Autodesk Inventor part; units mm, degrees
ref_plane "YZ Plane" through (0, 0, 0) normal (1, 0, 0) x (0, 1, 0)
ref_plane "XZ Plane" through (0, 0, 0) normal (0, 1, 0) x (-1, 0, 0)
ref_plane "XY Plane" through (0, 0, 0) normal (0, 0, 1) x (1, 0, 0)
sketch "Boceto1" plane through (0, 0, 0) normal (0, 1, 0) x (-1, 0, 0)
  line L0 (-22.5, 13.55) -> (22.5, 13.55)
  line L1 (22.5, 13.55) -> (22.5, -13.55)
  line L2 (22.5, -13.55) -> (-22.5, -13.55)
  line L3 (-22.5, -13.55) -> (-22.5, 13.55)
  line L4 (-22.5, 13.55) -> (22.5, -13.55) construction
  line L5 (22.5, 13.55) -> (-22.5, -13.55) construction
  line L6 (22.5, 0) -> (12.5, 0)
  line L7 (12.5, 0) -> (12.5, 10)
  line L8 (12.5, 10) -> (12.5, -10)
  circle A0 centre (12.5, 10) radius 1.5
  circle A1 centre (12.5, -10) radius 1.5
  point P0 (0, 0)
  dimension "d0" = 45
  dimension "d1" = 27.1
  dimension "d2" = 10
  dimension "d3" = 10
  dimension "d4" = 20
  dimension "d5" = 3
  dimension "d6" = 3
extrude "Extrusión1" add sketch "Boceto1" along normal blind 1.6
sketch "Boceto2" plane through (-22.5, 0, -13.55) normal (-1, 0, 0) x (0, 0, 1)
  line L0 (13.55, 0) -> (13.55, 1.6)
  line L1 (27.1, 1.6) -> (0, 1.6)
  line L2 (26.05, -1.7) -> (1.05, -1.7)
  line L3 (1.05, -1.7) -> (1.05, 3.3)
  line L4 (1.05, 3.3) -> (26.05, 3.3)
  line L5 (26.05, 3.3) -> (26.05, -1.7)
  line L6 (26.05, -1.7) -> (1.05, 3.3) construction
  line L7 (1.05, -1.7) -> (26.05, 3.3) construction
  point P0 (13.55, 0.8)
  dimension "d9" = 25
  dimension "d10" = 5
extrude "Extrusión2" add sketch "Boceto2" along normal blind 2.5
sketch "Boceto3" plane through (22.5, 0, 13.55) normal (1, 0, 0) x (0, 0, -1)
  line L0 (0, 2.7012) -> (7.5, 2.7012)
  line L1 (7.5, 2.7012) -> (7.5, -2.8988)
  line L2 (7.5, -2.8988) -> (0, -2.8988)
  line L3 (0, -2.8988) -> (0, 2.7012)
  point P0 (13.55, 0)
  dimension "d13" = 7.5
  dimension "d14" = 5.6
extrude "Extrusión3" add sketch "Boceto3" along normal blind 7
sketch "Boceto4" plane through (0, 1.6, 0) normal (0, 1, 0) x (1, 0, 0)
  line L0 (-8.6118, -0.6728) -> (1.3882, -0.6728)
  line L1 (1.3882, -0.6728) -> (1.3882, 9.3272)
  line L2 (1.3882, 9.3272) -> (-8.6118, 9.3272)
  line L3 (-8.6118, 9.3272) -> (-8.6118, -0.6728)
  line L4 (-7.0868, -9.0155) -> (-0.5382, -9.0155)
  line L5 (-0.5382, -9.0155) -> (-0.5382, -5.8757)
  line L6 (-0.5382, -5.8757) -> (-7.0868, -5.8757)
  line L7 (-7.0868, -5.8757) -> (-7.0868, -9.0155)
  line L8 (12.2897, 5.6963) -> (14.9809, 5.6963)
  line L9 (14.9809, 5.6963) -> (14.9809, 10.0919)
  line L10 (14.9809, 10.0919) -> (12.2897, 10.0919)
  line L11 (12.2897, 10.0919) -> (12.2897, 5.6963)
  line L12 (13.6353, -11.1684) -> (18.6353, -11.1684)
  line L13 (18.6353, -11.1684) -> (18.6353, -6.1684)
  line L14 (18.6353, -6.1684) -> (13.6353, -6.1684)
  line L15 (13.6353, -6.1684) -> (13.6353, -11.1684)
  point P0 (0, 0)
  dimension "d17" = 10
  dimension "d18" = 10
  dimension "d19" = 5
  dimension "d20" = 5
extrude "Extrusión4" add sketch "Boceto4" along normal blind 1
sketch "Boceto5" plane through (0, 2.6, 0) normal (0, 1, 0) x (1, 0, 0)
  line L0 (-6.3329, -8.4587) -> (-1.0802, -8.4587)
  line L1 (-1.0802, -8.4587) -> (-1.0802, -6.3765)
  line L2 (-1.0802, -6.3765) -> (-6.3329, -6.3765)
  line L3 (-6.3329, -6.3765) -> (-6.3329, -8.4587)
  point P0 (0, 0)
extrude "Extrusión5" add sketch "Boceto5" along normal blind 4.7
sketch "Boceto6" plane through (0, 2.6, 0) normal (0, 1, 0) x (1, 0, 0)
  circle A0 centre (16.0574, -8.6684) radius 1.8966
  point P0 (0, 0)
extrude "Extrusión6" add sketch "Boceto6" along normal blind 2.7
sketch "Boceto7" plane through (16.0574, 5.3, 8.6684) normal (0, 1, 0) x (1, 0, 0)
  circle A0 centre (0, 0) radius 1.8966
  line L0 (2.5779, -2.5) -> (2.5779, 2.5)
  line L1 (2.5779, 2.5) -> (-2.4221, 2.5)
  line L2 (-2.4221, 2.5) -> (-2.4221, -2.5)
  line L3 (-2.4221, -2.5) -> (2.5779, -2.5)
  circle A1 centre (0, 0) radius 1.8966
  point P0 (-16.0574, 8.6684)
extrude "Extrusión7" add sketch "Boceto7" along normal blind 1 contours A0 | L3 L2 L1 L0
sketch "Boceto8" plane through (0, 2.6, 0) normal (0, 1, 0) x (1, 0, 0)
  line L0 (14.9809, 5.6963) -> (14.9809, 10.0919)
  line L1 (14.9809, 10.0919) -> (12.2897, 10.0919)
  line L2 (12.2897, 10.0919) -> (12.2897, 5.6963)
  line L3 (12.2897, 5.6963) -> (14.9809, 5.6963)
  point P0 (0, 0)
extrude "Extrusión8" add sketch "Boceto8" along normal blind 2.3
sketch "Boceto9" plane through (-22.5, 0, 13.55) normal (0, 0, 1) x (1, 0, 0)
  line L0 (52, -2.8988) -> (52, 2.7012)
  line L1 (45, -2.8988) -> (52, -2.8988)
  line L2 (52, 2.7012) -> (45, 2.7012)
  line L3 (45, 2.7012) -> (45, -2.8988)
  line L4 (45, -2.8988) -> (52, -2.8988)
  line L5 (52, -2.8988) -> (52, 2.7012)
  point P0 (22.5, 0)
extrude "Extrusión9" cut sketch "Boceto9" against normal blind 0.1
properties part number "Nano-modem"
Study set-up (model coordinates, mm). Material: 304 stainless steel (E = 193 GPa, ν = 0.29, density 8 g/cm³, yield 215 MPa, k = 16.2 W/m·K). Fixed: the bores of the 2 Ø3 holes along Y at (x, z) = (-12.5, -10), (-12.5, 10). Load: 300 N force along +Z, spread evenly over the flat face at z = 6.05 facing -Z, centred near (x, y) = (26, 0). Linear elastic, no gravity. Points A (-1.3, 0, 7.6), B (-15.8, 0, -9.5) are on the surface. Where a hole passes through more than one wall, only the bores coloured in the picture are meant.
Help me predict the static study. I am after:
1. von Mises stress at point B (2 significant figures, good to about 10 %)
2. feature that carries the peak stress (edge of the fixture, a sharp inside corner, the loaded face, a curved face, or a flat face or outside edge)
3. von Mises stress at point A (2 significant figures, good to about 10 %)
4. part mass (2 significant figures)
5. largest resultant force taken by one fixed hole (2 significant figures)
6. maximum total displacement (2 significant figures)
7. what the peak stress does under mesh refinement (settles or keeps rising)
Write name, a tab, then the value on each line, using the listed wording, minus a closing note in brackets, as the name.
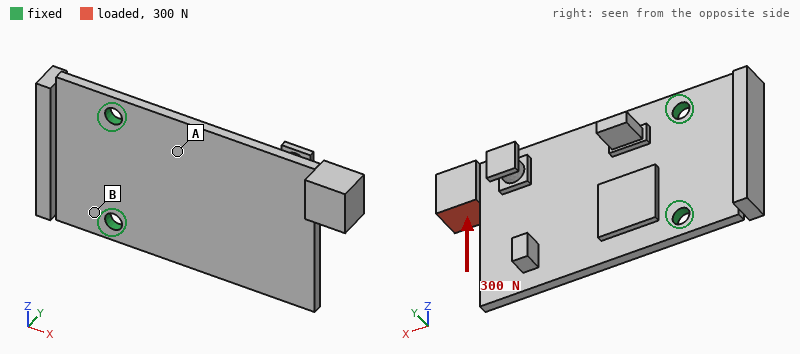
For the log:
von Mises stress at point B	10 MPa
feature that carries the peak stress	a sharp inside corner
von Mises stress at point A	33 MPa
part mass	23 g
largest resultant force taken by one fixed hole	570 N
maximum total displacement	57 µm
what the peak stress does under mesh refinement	keeps rising
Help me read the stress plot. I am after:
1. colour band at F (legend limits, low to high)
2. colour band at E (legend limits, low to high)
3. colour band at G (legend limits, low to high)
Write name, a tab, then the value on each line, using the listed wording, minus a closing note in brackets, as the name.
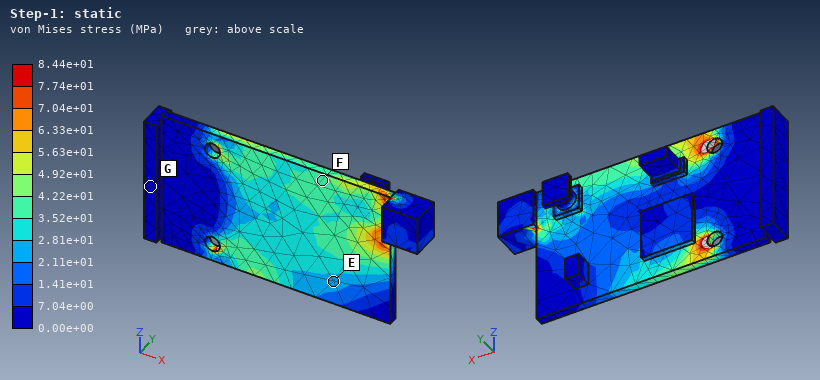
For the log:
colour band at F	3.52e+01 to 4.22e+01 MPa
colour band at E	2.11e+01 to 2.81e+01 MPa
colour band at G	0.00e+00 to 7.04e+00 MPa
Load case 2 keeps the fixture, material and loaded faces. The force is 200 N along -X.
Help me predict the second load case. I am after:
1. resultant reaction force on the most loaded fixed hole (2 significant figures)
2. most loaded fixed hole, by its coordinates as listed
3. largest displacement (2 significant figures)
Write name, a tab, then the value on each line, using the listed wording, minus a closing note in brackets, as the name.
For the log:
resultant reaction force on the most loaded fixed hole	160 N
most loaded fixed hole, by its coordinates as listed	(-12.5, 10)
largest displacement	86 µm
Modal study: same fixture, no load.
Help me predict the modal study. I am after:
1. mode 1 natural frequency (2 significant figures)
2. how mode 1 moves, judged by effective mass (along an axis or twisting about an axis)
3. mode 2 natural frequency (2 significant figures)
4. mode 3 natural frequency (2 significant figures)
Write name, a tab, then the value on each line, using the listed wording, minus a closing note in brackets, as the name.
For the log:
mode 1 natural frequency	790 Hz
how mode 1 moves, judged by effective mass	along Y
mode 2 natural frequency	2700 Hz
mode 3 natural frequency	4700 Hz
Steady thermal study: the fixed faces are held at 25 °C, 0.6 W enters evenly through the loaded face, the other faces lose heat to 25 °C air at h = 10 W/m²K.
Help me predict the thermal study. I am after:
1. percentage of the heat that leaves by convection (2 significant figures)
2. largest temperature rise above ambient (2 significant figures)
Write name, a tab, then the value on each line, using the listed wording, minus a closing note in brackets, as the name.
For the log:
percentage of the heat that leaves by convection	47 %
largest temperature rise above ambient	35 K
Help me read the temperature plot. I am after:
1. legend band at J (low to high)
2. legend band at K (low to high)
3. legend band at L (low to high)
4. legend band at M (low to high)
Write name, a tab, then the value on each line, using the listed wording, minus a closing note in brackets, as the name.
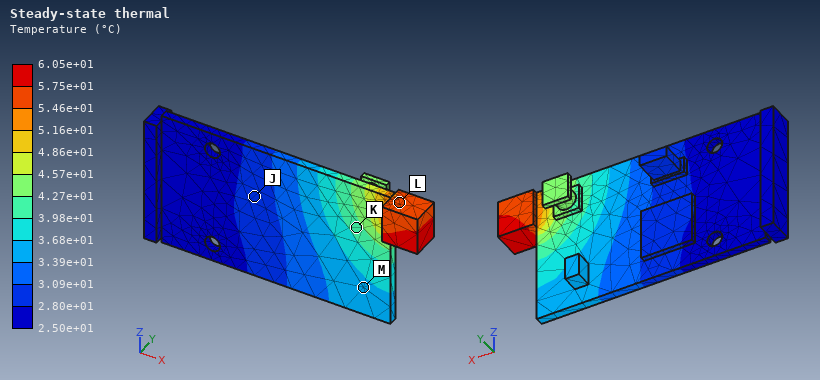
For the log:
legend band at J	2.80e+01 to 3.09e+01 °C
legend band at K	3.98e+01 to 4.27e+01 °C
legend band at L	5.46e+01 to 5.75e+01 °C
legend band at M	3.39e+01 to 3.68e+01 °C
